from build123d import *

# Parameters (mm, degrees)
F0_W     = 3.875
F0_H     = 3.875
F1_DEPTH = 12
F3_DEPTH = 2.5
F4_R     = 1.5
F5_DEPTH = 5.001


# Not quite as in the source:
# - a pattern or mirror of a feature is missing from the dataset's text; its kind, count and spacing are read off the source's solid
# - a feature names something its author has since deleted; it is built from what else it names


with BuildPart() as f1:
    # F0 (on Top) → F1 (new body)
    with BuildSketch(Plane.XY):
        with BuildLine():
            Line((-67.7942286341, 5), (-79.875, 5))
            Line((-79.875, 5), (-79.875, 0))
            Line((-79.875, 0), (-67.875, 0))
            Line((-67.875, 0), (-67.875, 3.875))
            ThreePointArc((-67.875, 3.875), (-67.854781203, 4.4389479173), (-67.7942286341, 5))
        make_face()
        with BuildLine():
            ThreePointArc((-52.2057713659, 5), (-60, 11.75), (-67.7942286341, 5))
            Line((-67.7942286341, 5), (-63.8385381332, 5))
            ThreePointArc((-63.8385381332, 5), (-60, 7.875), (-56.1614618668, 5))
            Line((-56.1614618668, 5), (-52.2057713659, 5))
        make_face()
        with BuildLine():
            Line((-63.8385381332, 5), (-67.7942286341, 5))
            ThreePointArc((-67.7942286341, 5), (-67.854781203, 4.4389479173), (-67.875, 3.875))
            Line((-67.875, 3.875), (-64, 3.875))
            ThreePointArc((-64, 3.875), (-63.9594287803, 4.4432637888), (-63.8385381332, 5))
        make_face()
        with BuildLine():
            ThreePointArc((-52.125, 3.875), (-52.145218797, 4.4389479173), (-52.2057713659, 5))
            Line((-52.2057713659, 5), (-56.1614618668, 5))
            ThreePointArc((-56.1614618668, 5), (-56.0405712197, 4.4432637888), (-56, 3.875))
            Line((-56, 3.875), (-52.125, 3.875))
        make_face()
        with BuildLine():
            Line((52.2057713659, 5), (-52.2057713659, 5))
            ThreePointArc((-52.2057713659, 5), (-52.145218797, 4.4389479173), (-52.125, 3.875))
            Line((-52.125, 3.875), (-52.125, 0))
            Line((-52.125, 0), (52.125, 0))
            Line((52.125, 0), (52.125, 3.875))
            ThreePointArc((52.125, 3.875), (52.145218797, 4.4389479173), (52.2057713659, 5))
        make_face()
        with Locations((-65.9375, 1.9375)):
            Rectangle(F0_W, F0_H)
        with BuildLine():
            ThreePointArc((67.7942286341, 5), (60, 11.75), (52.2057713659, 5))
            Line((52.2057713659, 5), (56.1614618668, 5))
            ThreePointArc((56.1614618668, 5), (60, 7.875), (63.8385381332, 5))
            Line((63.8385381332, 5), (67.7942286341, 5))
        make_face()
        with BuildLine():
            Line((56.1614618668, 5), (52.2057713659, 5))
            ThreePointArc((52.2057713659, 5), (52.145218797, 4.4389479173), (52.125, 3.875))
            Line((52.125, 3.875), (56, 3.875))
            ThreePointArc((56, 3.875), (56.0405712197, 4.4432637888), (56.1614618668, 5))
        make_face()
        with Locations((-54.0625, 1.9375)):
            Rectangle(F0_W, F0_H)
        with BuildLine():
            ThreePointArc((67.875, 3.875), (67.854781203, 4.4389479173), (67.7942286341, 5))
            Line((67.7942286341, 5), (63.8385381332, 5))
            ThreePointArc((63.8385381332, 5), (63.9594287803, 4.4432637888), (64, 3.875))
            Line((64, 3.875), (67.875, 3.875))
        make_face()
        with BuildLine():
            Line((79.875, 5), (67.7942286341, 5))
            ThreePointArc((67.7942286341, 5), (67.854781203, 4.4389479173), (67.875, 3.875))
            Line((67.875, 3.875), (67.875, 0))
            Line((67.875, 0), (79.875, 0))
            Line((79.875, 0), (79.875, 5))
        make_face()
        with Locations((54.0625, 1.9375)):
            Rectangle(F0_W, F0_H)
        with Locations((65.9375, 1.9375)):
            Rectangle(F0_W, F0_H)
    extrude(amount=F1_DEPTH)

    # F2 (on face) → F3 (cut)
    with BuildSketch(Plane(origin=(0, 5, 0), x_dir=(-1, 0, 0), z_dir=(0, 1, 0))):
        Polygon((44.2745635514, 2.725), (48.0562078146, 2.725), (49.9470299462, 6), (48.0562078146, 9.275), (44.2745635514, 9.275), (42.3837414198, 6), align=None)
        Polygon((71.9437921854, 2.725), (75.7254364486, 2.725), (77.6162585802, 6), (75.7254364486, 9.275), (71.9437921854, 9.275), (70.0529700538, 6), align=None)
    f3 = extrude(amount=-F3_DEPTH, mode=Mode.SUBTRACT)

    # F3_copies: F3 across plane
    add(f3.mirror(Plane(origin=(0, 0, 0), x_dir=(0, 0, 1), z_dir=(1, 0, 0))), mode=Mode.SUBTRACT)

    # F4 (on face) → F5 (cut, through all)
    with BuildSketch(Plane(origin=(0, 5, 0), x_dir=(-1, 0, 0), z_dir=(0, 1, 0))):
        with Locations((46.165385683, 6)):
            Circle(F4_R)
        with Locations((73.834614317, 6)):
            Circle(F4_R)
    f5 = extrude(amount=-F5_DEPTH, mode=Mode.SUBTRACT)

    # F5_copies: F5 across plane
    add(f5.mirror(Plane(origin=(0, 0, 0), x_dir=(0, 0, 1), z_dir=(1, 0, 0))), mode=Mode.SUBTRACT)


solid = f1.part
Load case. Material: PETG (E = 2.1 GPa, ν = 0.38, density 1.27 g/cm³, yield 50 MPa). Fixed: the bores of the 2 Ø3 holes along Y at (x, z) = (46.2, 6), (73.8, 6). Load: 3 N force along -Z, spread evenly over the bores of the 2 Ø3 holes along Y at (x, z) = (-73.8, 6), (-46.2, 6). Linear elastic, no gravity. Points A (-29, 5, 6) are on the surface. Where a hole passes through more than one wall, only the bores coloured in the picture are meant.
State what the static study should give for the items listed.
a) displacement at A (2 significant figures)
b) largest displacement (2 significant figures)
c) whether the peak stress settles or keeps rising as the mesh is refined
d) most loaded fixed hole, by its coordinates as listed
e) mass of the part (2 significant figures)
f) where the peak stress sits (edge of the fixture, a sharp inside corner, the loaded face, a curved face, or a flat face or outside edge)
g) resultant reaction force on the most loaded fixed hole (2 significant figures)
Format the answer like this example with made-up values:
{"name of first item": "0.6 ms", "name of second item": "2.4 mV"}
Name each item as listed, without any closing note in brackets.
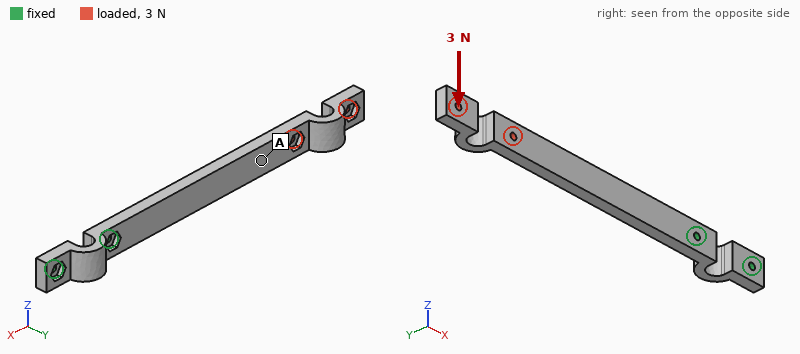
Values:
{"displacement at A": "0.68 mm", "largest displacement": "1.4 mm", "whether the peak stress settles or keeps rising as the mesh is refined": "keeps rising", "most loaded fixed hole, by its coordinates as listed": "(46.2, 6)", "mass of the part": "12 g", "where the peak stress sits": "edge of the fixture", "resultant reaction force on the most loaded fixed hole": "9.1 N"}
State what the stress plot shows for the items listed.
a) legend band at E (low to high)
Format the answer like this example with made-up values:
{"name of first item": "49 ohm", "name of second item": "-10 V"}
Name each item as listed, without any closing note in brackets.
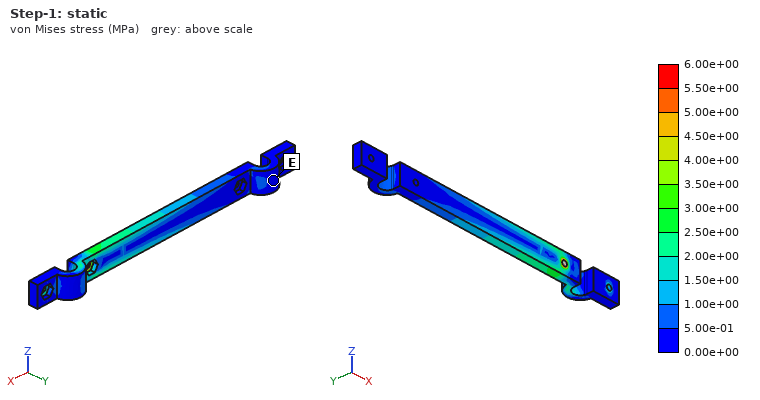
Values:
{"legend band at E": "0.00e+00 to 5.00e-01 MPa"}
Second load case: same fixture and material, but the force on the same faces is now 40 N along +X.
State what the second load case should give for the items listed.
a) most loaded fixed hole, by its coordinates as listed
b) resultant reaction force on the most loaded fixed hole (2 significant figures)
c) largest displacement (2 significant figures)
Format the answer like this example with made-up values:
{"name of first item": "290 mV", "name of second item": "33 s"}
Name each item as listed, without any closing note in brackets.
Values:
{"most loaded fixed hole, by its coordinates as listed": "(46.2, 6)", "resultant reaction force on the most loaded fixed hole": "39 N", "largest displacement": "1.8 mm"}
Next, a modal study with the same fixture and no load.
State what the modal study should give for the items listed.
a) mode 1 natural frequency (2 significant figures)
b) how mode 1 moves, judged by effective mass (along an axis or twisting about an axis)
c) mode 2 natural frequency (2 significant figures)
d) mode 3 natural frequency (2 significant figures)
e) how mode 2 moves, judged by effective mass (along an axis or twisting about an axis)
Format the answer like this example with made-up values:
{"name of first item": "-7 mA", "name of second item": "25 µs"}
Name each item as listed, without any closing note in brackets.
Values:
{"mode 1 natural frequency": "60 Hz", "how mode 1 moves, judged by effective mass": "along Y", "mode 2 natural frequency": "130 Hz", "mode 3 natural frequency": "370 Hz", "how mode 2 moves, judged by effective mass": "along Z"}
